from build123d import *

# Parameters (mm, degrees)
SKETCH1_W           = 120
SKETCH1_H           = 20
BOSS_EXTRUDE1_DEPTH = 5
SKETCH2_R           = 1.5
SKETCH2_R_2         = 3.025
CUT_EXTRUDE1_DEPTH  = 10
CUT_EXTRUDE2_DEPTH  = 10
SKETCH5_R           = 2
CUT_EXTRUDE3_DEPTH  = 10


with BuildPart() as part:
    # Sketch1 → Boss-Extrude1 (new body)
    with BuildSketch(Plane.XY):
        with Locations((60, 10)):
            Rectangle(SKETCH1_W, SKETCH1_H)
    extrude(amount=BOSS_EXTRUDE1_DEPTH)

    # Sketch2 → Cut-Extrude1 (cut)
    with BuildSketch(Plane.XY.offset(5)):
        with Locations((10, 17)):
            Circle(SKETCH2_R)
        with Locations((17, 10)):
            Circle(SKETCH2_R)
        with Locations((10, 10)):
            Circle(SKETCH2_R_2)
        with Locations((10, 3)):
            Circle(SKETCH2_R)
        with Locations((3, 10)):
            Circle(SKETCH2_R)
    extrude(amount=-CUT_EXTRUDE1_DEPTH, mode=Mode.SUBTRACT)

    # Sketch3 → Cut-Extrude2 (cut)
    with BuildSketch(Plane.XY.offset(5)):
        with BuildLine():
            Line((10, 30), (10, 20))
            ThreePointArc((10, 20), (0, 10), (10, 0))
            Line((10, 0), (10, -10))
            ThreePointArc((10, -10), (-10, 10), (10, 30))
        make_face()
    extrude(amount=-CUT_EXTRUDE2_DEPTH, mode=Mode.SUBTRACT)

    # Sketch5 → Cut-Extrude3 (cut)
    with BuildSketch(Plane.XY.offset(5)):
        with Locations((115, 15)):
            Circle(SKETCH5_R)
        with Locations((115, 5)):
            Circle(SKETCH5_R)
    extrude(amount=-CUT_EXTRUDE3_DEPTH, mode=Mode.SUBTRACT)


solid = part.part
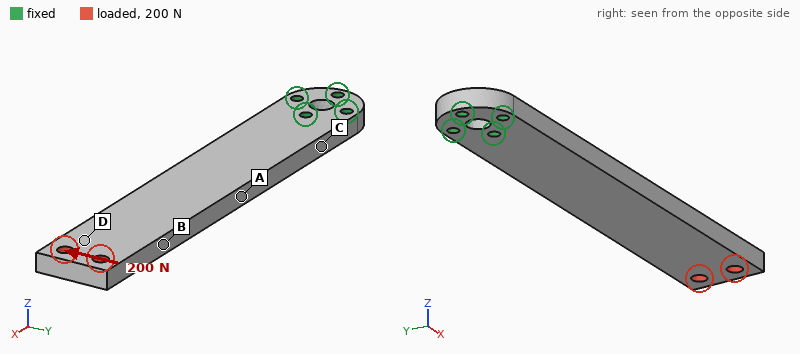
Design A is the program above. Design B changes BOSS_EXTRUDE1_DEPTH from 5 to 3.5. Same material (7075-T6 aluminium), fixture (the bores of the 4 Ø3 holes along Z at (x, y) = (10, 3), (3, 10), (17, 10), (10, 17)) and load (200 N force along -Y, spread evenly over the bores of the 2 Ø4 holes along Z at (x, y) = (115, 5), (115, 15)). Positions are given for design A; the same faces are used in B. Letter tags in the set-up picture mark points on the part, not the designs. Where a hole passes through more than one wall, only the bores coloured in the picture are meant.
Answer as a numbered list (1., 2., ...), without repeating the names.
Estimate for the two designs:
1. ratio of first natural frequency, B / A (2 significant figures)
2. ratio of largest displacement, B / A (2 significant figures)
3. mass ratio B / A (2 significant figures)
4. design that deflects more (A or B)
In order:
1. 0.71
2. 1.4
3. 0.70
4. B
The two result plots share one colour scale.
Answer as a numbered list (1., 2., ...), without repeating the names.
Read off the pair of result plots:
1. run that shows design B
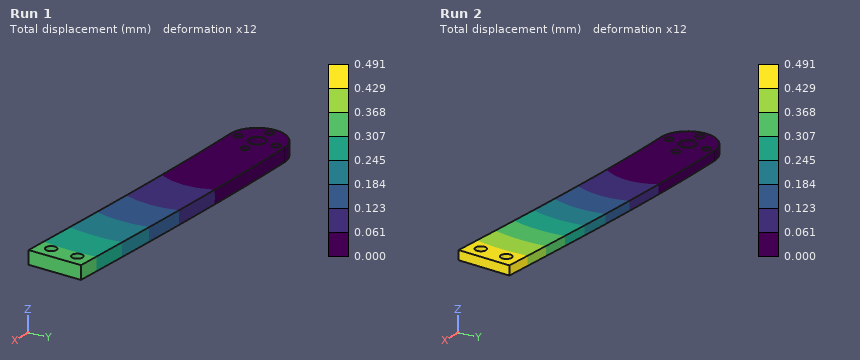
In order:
1. Run 2
